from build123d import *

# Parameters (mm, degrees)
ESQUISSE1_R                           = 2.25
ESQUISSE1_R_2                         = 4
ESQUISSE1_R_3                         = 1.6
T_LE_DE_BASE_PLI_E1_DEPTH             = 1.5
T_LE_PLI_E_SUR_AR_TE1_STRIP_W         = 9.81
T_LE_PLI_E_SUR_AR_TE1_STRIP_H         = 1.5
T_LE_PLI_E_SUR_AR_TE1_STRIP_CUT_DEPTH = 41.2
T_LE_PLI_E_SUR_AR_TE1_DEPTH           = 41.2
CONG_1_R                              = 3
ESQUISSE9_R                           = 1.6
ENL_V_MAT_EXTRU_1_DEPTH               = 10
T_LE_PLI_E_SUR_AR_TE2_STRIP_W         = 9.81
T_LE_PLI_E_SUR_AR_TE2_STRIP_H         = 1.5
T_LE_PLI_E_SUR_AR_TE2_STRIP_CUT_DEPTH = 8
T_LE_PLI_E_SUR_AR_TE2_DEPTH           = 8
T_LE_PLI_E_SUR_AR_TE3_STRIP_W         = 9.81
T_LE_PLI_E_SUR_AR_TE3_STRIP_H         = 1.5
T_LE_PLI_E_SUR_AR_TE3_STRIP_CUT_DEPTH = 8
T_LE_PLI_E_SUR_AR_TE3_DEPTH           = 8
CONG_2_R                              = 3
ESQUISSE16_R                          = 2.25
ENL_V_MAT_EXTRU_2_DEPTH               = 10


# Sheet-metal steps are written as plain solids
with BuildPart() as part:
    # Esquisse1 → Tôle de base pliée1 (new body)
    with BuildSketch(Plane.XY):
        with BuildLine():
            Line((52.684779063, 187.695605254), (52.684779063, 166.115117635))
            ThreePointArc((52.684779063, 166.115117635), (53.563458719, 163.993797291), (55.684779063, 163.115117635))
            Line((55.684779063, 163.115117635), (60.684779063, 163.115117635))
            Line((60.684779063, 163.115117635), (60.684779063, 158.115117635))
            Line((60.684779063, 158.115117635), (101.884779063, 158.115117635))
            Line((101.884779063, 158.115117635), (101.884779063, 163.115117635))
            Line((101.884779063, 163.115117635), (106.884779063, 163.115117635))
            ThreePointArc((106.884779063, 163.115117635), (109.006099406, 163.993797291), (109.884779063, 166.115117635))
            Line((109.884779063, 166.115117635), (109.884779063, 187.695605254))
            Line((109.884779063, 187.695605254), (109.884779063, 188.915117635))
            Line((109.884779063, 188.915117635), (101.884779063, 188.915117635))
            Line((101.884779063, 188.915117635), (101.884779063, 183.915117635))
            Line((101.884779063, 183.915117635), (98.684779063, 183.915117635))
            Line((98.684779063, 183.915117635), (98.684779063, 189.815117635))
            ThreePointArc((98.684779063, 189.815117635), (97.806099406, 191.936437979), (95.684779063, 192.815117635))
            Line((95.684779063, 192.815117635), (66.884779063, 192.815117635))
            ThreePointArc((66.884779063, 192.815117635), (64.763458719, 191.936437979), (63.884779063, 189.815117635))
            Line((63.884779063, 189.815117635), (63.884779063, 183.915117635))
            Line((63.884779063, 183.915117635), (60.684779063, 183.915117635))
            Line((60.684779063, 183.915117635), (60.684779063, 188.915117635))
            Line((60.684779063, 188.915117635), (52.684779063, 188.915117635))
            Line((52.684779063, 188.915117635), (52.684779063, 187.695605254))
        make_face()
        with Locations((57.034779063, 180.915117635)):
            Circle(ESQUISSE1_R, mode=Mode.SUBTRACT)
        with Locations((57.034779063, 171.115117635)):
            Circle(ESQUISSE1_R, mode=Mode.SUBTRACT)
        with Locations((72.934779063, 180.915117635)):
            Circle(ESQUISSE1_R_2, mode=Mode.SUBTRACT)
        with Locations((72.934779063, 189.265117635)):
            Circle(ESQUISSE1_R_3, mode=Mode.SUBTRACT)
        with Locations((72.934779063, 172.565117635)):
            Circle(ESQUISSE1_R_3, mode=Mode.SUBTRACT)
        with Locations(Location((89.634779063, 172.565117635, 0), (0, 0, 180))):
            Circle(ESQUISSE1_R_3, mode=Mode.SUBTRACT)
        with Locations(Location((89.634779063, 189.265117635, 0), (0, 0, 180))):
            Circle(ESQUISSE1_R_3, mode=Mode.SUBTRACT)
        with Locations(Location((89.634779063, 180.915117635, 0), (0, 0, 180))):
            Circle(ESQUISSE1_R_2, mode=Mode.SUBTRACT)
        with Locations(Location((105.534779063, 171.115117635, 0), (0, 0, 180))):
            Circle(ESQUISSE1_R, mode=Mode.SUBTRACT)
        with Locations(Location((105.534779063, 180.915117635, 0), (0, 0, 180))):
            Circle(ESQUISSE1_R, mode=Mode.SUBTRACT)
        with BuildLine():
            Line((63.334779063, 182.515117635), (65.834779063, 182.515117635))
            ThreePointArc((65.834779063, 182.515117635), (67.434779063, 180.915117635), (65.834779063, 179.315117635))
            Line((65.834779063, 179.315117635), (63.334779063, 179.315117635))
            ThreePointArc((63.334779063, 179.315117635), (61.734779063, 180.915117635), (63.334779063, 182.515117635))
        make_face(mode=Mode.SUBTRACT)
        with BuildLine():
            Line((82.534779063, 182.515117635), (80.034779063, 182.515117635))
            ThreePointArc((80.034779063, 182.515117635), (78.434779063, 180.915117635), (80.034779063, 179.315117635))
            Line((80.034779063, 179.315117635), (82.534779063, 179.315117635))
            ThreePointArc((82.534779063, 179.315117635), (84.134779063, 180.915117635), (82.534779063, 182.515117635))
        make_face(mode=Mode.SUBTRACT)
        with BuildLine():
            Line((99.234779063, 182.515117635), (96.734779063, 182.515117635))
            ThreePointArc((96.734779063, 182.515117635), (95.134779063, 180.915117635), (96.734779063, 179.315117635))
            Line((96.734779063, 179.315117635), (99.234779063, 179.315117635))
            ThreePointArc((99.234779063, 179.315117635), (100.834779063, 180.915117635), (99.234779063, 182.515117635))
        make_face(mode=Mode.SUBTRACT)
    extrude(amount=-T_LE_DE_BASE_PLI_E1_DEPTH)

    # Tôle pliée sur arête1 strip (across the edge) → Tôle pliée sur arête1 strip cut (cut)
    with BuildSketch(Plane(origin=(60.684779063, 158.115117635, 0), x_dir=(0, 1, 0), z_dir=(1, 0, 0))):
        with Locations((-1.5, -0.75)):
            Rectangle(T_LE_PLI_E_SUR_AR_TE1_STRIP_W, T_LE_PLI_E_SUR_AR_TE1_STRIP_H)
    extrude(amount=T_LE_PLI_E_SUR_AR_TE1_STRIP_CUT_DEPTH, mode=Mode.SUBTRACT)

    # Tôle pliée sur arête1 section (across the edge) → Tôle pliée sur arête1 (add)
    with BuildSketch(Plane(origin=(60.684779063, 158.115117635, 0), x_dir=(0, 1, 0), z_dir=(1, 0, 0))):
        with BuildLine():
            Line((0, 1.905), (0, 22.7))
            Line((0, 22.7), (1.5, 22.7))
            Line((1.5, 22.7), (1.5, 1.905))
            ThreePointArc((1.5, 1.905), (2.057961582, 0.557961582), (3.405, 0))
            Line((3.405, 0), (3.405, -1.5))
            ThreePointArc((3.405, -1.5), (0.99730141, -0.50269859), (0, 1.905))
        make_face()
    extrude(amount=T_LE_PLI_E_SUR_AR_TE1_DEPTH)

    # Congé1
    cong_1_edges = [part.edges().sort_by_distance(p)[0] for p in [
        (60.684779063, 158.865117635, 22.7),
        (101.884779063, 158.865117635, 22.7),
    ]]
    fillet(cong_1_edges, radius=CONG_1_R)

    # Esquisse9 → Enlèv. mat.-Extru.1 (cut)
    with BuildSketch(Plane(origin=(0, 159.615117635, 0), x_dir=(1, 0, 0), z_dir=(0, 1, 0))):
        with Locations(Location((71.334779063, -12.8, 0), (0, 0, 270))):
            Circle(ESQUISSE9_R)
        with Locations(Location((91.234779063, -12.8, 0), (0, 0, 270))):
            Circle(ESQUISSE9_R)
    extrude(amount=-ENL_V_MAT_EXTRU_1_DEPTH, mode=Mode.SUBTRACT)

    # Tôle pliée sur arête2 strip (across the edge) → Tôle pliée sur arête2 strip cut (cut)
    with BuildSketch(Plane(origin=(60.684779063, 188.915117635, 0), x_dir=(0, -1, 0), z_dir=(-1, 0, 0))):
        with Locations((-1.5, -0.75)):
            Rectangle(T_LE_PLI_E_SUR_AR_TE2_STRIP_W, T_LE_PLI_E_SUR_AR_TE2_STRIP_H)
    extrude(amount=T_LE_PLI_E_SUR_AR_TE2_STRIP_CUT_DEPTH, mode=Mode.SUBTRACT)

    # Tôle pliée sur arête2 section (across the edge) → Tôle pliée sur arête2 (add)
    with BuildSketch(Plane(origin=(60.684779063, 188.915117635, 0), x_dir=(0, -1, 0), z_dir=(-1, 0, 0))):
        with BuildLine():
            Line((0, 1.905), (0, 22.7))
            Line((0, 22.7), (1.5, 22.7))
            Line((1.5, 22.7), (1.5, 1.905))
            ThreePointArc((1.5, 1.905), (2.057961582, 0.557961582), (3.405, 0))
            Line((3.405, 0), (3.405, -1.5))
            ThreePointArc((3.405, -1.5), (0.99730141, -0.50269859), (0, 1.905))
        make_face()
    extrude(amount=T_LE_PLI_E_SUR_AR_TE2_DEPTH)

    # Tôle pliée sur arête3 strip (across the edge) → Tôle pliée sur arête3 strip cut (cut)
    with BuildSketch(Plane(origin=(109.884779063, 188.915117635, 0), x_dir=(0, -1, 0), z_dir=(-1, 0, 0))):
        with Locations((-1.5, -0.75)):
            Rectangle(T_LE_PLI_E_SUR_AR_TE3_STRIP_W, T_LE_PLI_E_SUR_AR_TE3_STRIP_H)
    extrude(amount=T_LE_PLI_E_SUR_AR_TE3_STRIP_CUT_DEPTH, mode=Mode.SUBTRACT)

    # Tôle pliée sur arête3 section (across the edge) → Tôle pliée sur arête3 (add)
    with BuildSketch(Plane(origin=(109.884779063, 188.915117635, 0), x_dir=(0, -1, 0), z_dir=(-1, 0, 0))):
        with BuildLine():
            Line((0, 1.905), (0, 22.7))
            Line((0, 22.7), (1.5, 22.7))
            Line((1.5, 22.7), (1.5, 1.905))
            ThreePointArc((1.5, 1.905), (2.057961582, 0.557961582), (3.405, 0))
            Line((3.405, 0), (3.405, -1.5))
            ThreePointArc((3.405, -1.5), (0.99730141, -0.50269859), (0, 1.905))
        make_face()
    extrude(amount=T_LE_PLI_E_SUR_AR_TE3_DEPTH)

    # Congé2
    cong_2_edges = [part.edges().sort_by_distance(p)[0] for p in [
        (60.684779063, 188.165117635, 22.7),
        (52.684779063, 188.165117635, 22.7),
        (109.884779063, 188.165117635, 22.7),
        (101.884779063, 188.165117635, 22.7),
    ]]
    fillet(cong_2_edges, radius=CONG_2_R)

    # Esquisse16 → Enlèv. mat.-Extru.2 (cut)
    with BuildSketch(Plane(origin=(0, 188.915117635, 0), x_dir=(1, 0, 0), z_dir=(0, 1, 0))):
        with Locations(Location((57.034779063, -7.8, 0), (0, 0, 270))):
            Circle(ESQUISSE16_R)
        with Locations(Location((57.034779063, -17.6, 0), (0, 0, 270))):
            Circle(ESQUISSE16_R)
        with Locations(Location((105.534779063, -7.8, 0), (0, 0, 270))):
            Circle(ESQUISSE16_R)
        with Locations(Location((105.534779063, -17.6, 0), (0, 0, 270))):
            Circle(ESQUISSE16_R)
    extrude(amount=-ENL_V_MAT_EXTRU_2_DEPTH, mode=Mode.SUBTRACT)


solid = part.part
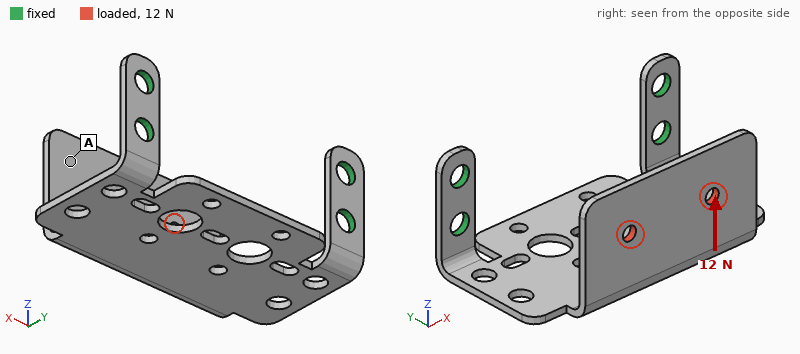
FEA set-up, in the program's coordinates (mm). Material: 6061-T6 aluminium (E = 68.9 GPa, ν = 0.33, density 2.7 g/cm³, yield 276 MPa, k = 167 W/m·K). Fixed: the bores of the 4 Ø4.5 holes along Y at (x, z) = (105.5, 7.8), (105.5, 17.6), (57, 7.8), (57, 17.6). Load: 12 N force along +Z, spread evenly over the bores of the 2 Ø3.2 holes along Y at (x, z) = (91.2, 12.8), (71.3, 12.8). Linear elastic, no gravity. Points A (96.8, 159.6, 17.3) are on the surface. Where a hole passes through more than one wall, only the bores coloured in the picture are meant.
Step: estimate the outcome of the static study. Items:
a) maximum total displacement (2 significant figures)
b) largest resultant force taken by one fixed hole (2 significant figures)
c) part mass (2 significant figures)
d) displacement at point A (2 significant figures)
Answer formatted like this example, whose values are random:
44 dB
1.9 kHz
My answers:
0.68 mm
6.1 N
11 g
0.59 mm
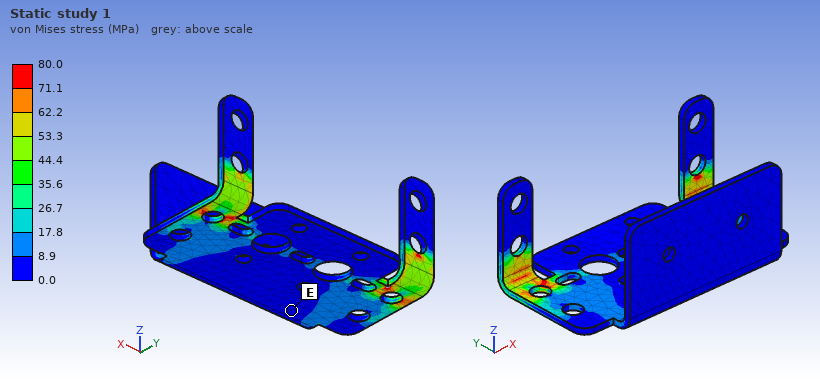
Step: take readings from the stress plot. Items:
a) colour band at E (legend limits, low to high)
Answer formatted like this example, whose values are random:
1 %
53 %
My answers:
0.0 to 8.9 MPa
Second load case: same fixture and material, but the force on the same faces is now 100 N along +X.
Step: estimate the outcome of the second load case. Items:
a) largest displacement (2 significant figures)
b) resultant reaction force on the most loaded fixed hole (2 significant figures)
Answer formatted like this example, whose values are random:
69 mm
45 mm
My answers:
0.73 mm
82 N
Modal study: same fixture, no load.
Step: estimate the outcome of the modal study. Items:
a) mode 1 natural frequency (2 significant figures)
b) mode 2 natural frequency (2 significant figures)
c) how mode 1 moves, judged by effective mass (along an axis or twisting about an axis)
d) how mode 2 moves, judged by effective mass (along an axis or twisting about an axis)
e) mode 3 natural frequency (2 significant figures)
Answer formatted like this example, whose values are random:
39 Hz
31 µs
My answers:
310 Hz
970 Hz
along Z
along X
1300 Hz
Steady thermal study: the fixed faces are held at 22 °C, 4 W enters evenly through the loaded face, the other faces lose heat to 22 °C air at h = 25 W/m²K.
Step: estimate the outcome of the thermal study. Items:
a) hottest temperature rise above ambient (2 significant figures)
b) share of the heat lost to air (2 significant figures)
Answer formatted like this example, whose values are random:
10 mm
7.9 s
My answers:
21 K
48 %
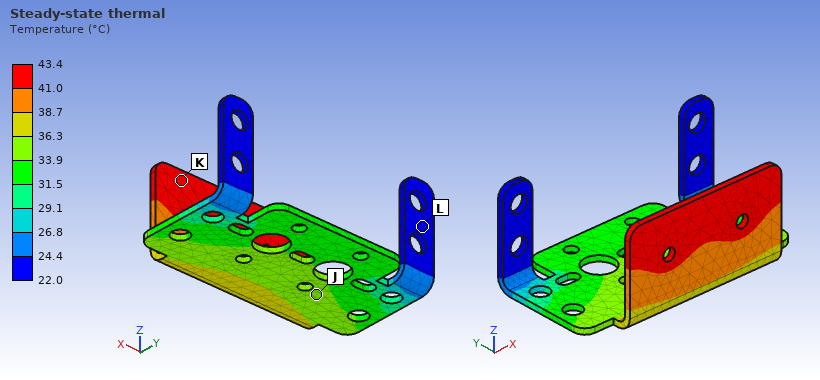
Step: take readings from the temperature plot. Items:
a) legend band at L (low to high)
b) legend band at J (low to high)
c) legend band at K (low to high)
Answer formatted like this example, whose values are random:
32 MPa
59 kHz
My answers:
22.0 to 24.4 °C
33.9 to 36.3 °C
41.0 to 43.4 °C
